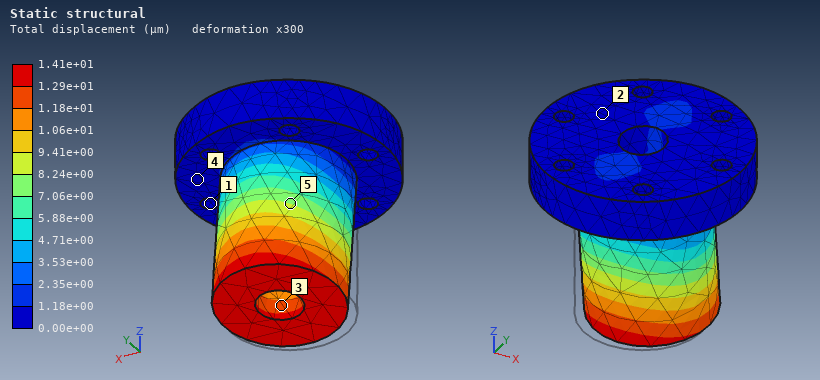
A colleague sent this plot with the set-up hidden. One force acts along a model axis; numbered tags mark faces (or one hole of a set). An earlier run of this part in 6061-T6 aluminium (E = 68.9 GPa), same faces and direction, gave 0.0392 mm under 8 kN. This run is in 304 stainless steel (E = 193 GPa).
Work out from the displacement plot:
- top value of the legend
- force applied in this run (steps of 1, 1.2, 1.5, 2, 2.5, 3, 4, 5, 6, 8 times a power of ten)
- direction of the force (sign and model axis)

1.41e+01 µm
8 kN
+Y
